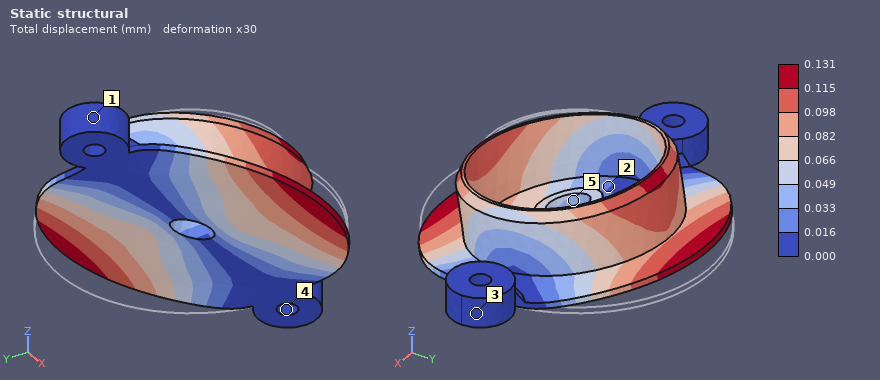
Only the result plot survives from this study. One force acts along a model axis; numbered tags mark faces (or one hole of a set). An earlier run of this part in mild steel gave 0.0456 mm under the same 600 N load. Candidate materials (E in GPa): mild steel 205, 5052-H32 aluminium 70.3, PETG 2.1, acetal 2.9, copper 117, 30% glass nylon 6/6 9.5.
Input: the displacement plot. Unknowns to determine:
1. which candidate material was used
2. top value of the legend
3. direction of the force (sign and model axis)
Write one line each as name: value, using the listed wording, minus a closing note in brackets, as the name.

which candidate material was used: 5052-H32 aluminium
top value of the legend: 0.131 mm
direction of the force: -Y
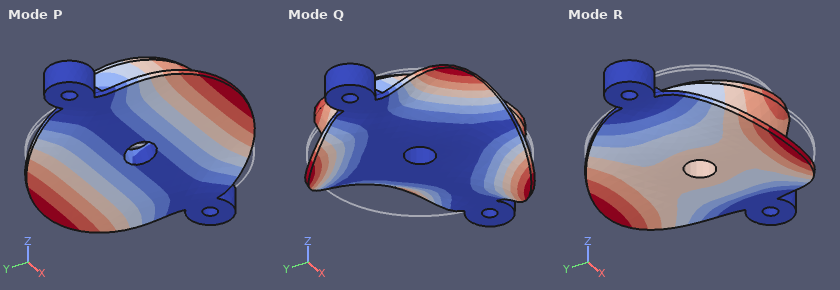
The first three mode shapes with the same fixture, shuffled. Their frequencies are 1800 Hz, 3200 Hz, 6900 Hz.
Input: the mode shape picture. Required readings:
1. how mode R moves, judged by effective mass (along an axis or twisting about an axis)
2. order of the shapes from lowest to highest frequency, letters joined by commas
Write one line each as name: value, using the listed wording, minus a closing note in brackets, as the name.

how mode R moves, judged by effective mass: along Z
order of the shapes from lowest to highest frequency, letters joined by commas: P, R, Q
